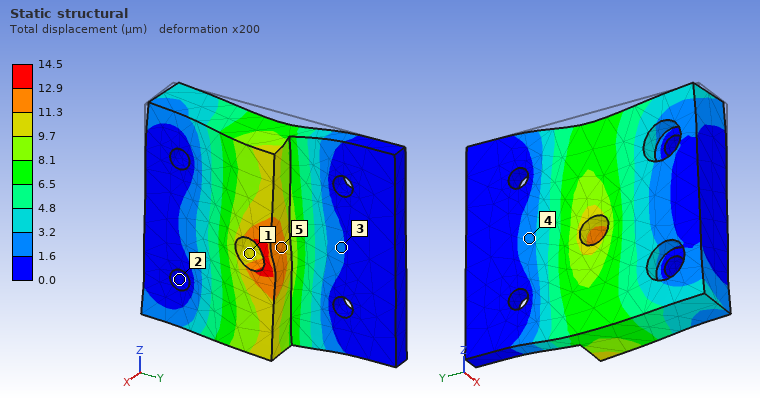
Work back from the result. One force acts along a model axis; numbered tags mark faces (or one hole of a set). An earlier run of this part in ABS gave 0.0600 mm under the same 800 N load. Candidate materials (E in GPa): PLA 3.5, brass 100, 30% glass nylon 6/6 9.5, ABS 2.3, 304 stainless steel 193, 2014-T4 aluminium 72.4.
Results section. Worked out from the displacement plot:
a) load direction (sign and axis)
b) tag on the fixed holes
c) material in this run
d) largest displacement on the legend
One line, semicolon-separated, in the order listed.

-Z; 2; 30% glass nylon 6/6; 14.5 µm
